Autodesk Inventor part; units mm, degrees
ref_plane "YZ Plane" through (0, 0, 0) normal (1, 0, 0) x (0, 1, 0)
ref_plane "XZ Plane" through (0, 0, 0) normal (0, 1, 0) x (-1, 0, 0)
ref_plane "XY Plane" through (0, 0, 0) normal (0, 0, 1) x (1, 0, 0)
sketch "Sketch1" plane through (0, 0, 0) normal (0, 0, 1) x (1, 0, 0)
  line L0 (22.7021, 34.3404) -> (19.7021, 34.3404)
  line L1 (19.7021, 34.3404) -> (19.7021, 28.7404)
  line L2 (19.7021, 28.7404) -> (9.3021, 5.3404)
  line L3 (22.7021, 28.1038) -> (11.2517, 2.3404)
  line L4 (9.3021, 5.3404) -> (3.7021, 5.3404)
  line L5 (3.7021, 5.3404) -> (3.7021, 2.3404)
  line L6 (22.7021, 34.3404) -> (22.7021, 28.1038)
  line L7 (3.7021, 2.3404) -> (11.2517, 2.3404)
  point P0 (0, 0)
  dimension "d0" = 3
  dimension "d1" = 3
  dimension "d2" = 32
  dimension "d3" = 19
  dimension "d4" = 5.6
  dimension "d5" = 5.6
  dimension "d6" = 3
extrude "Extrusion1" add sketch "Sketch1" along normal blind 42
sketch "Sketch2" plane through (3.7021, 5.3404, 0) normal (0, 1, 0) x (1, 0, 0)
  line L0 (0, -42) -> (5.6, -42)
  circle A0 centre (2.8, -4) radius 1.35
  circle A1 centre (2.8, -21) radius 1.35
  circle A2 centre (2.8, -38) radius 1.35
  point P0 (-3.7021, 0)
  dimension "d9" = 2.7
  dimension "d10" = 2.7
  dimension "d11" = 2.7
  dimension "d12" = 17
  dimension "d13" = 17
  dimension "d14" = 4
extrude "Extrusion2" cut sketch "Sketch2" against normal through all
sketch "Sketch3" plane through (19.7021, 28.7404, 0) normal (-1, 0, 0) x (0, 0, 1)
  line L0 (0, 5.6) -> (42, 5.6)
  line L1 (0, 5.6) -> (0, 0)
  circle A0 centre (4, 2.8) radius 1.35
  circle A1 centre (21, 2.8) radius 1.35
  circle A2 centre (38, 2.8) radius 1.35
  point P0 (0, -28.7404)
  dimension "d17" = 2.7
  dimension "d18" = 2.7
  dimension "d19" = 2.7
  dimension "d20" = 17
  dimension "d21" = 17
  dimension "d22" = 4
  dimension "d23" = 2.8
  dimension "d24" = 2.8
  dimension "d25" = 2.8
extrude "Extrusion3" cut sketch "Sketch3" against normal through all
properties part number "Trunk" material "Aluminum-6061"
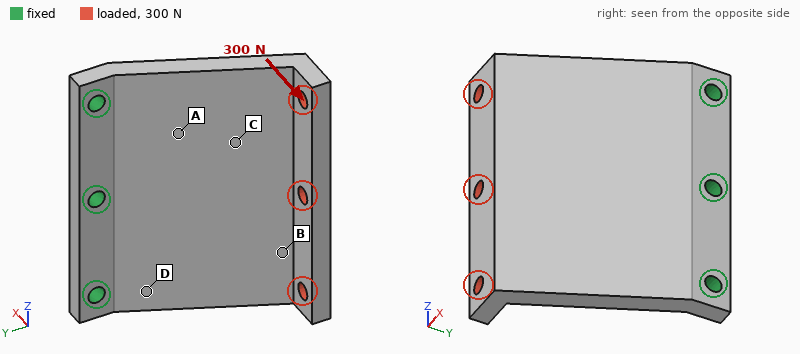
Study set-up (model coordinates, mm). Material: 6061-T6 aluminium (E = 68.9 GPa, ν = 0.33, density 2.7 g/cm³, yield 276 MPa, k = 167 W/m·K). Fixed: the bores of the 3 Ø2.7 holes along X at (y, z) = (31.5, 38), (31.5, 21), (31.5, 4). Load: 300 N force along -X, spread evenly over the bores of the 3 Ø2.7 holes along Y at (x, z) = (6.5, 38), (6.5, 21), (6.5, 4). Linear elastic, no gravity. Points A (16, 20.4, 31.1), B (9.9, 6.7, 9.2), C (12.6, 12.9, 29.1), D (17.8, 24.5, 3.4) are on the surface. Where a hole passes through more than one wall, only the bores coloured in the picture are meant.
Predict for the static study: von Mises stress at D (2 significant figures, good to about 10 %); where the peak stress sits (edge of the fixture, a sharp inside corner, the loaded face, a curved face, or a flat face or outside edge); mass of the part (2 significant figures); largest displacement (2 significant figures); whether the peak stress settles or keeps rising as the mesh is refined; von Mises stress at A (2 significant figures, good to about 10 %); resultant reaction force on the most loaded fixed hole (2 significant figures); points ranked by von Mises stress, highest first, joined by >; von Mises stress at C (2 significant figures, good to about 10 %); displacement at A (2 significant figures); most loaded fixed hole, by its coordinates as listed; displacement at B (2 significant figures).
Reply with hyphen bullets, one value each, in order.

- 91 MPa
- edge of the fixture
- 13 g
- 0.48 mm
- keeps rising
- 70 MPa
- 170 N
- D > A > C > B
- 36 MPa
- 0.097 mm
- (31.5, 21)
- 0.34 mm
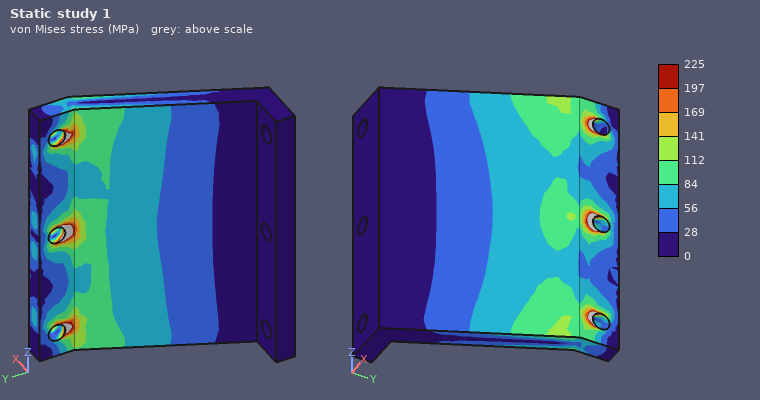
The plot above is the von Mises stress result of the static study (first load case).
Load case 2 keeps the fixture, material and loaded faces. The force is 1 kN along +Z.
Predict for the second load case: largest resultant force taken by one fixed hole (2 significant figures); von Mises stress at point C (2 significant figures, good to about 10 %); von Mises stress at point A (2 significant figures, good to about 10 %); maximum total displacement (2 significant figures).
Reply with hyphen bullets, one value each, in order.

- 940 N
- 55 MPa
- 52 MPa
- 0.17 mm
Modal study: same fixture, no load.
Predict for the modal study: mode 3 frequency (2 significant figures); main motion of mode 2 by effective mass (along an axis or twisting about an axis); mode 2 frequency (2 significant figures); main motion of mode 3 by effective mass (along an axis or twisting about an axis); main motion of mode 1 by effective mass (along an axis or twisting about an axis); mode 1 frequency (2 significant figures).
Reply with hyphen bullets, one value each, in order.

- 11 kHz
- twisting about Y
- 4100 Hz
- along X
- along X
- 1900 Hz
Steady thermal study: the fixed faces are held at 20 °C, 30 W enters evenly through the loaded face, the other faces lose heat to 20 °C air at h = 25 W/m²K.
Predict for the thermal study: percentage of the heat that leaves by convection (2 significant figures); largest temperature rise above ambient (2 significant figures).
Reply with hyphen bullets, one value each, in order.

- 7.6 %
- 54 K
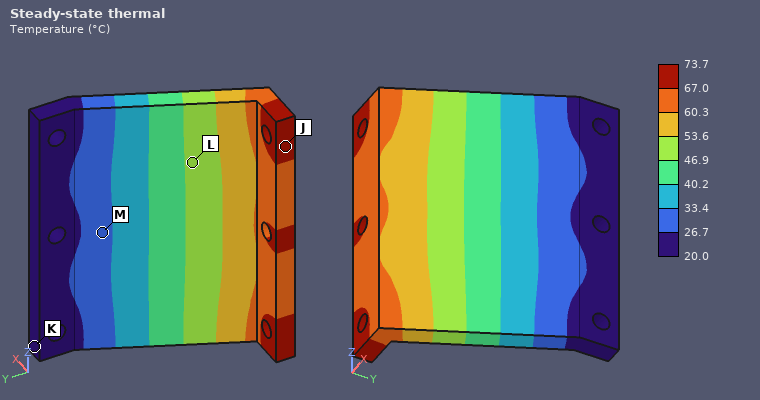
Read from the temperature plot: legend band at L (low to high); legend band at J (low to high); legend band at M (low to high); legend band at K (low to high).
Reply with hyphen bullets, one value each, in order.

- 46.9 to 53.6 °C
- 67.0 to 73.7 °C
- 26.7 to 33.4 °C
- 20.0 to 26.7 °C
